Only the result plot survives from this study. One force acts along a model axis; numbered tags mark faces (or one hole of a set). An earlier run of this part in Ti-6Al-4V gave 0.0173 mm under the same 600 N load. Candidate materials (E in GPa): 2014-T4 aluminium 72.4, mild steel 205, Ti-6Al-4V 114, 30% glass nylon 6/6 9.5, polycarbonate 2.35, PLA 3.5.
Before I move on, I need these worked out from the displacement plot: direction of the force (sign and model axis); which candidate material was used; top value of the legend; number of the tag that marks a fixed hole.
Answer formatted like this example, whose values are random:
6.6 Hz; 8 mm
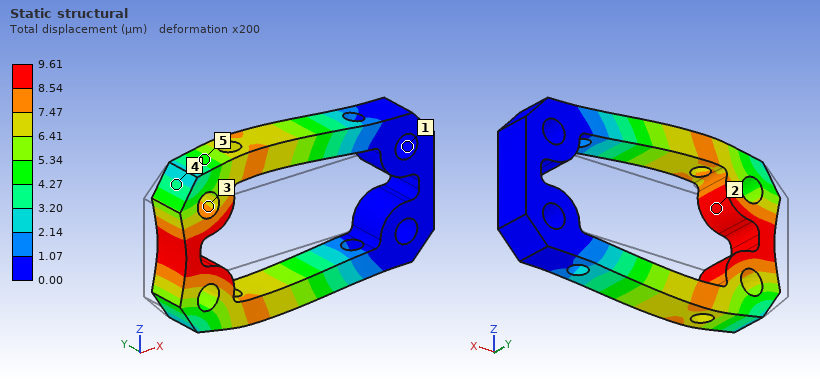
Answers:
+X; mild steel; 9.61 µm; 1
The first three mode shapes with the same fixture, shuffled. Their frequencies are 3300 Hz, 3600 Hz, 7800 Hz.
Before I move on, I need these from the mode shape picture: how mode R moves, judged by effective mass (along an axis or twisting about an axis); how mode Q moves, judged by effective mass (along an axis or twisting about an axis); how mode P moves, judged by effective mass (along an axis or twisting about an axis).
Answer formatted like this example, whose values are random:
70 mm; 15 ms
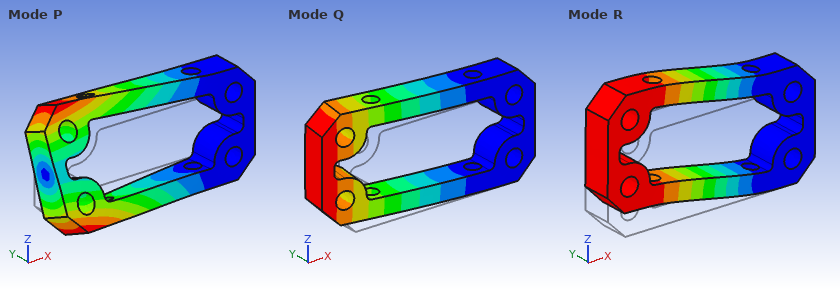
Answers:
along Z; along Y; twisting about X
